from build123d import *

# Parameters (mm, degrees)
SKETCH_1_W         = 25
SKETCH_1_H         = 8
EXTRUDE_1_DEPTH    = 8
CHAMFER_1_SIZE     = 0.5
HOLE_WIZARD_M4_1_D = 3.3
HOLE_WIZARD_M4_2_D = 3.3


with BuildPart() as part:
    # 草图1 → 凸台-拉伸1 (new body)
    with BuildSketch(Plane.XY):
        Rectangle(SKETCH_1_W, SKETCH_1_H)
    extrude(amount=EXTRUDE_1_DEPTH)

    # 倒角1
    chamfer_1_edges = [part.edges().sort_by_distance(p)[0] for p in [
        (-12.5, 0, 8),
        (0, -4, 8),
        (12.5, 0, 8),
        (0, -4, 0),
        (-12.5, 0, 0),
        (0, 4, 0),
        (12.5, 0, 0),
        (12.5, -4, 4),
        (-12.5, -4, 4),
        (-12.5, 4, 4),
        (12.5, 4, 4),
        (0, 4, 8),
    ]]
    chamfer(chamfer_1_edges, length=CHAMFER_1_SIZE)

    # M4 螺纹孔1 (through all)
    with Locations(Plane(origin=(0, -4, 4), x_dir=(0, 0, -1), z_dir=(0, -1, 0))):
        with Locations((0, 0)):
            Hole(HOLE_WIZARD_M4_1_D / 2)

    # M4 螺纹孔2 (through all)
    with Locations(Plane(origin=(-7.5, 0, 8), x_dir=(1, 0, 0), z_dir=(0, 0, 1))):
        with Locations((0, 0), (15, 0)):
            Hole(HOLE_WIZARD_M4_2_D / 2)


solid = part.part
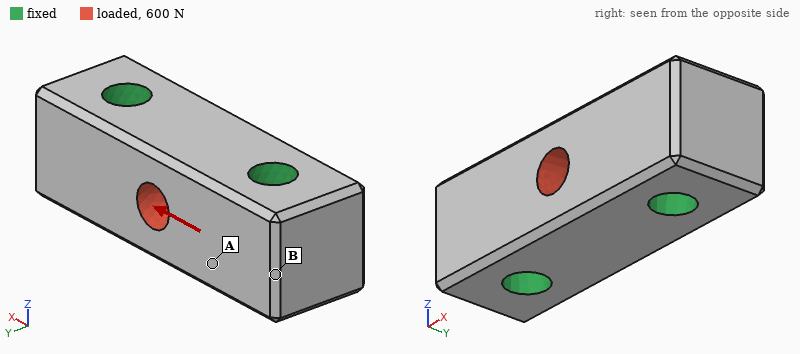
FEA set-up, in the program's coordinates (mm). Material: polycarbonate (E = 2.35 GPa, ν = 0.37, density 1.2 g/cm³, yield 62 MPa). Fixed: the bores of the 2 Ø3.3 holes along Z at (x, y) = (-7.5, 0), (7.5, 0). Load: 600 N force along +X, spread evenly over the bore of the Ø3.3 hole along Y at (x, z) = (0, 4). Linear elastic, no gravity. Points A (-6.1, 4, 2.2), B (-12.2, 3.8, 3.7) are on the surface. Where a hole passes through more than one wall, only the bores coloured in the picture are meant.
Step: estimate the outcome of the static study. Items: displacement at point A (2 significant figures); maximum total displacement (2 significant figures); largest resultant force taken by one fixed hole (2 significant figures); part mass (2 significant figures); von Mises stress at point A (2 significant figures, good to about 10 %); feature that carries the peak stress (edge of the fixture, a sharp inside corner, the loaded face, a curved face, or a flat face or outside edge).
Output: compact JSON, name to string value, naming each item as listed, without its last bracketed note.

{"displacement at point A": "5.7 µm", "maximum total displacement": "16 µm", "largest resultant force taken by one fixed hole": "300 N", "part mass": "1.6 g", "von Mises stress at point A": "2.5 MPa", "feature that carries the peak stress": "the loaded face"}
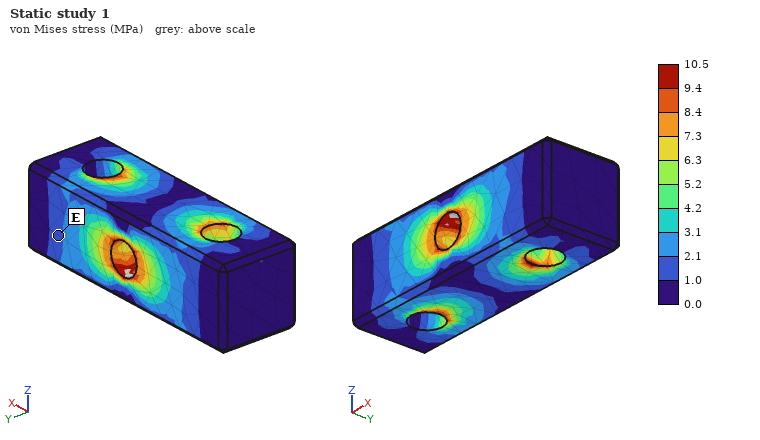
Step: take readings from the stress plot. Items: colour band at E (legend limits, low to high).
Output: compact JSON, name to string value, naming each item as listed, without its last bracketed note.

{"colour band at E": "1.0 to 2.1 MPa"}
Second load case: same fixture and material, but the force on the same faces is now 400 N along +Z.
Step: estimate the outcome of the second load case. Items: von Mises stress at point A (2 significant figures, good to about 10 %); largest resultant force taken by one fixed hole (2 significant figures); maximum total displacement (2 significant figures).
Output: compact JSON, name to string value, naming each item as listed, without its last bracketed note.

{"von Mises stress at point A": "2.8 MPa", "largest resultant force taken by one fixed hole": "200 N", "maximum total displacement": "34 µm"}
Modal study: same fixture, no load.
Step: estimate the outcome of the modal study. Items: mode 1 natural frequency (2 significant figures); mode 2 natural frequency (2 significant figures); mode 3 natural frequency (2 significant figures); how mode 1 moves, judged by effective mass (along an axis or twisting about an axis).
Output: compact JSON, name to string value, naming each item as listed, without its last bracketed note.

{"mode 1 natural frequency": "25 kHz", "mode 2 natural frequency": "29 kHz", "mode 3 natural frequency": "30 kHz", "how mode 1 moves, judged by effective mass": "along Y"}
